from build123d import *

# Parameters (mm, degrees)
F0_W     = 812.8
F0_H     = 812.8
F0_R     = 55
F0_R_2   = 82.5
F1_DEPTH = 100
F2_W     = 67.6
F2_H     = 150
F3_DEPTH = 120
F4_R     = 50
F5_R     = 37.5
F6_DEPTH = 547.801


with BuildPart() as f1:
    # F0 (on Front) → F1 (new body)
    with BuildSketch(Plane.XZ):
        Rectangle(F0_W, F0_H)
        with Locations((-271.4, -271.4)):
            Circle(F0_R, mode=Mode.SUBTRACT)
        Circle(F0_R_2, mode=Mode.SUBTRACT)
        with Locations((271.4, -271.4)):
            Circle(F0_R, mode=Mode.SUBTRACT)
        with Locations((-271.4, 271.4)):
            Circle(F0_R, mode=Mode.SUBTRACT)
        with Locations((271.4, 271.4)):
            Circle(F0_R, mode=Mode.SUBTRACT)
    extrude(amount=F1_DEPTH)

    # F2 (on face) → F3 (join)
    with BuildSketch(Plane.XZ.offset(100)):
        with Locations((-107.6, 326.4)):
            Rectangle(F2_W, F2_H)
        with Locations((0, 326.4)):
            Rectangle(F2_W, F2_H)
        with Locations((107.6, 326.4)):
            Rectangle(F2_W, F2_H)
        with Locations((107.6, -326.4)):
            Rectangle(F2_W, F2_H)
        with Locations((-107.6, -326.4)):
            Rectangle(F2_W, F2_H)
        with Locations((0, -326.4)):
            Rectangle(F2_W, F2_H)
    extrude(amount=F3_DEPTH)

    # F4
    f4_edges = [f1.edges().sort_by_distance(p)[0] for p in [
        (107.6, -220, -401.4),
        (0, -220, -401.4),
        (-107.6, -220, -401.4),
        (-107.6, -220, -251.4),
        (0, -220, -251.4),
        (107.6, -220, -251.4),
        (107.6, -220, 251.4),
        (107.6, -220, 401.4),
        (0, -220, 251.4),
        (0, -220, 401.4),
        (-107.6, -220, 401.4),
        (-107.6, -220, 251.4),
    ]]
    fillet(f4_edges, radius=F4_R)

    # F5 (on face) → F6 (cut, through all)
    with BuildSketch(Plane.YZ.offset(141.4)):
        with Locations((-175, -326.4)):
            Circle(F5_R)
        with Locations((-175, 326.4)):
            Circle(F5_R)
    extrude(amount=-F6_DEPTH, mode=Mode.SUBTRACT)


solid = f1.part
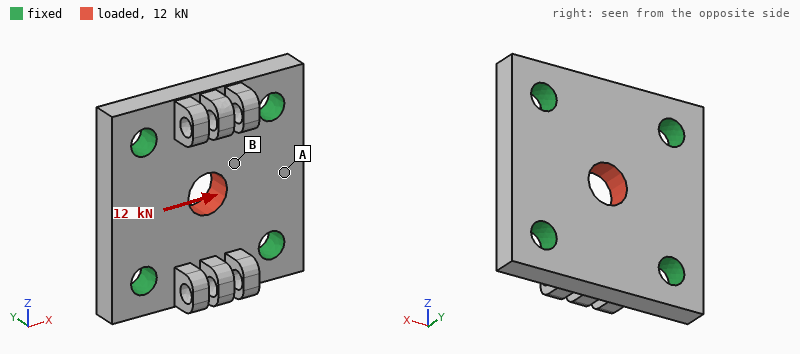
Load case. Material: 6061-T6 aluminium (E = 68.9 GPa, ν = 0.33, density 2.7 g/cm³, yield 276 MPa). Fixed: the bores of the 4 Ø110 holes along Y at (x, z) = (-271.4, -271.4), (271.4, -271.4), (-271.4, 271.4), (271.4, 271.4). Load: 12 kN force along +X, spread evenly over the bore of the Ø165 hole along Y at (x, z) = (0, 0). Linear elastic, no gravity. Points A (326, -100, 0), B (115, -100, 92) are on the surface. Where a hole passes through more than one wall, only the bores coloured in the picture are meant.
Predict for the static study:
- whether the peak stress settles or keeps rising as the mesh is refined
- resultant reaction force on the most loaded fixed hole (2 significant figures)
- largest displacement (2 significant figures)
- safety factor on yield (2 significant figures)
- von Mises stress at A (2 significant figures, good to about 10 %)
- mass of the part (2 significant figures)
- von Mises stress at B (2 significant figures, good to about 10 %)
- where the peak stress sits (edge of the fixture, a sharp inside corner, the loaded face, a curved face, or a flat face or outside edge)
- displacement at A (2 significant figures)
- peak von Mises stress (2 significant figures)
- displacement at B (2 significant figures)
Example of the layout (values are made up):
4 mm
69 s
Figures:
settles
3.3 kN
0.94 µm
670
0.045 MPa
180 kg
0.18 MPa
the loaded face
0.54 µm
0.41 MPa
0.61 µm
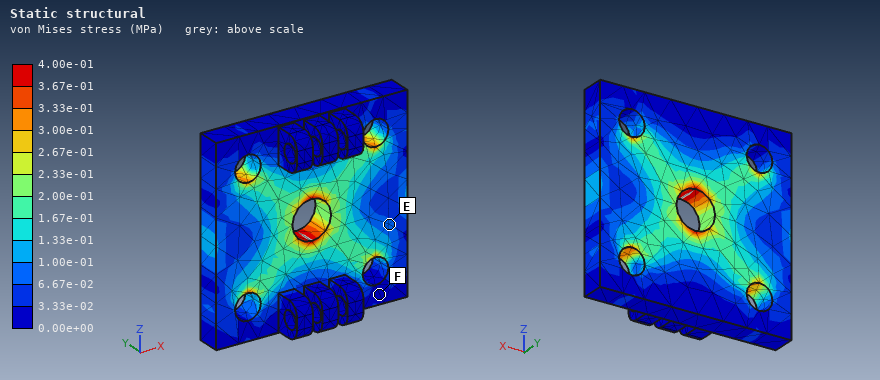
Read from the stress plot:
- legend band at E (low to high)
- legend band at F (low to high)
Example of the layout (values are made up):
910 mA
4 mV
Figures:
6.67e-02 to 1.00e-01 MPa
0.00e+00 to 3.33e-02 MPa
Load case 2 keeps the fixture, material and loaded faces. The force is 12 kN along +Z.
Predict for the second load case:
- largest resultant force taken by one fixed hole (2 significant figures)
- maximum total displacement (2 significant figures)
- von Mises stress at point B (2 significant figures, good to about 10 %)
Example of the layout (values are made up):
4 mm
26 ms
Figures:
3.3 kN
0.93 µm
0.17 MPa
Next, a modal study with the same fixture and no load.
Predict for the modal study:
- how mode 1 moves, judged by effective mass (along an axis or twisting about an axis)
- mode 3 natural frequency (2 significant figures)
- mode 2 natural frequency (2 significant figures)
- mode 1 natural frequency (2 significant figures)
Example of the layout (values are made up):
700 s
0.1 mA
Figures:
along Y
1500 Hz
1500 Hz
1300 Hz
